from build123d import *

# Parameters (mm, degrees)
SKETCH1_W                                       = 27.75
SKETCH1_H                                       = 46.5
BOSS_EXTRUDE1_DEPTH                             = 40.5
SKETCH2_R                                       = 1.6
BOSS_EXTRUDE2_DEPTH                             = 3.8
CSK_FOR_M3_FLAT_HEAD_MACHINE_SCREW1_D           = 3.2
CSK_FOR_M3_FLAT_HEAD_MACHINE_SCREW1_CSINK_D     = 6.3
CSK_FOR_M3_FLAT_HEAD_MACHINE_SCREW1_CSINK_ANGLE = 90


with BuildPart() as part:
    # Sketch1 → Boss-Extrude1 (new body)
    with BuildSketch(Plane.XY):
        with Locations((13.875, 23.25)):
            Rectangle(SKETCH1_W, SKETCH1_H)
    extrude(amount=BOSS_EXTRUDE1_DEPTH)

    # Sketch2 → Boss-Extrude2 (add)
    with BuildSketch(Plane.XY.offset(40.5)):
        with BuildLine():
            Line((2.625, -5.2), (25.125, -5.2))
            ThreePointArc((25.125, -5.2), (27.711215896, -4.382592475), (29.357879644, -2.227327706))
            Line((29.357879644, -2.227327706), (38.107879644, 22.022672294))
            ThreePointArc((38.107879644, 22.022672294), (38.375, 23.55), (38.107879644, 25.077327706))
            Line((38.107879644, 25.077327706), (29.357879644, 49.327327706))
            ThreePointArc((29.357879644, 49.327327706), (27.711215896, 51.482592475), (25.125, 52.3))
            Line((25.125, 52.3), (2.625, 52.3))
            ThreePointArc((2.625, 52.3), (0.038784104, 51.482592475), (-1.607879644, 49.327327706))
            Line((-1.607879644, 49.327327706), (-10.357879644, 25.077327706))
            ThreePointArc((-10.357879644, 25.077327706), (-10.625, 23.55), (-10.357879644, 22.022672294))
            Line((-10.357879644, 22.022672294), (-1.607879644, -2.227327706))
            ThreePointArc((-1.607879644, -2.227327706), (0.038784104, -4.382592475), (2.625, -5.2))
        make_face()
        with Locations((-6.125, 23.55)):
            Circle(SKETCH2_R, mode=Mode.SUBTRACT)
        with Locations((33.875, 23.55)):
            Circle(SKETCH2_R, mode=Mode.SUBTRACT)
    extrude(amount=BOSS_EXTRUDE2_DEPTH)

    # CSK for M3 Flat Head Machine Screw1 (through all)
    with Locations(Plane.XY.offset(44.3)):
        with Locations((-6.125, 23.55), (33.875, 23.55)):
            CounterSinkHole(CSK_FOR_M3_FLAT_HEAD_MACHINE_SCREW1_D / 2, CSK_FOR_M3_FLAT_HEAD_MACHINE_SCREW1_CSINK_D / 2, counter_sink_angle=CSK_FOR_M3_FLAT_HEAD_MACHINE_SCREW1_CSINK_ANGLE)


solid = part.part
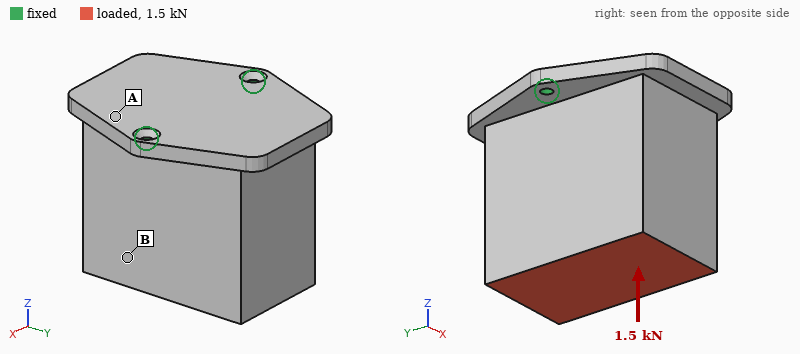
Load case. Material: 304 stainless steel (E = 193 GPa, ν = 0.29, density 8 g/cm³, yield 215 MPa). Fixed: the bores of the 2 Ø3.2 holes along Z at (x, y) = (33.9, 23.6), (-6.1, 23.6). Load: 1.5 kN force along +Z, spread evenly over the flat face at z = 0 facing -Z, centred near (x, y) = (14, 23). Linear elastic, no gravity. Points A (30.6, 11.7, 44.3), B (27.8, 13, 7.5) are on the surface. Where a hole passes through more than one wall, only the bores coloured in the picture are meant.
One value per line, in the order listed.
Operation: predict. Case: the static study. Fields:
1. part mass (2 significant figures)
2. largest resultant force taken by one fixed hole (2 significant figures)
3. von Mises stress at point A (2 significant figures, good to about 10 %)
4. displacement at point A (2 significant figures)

490 g
750 N
21 MPa
6.0 µm
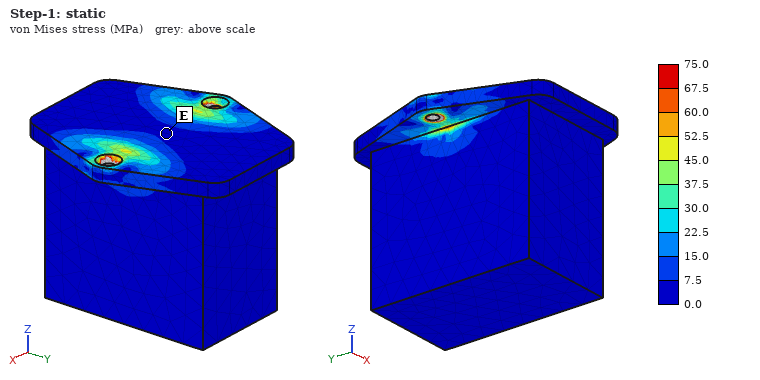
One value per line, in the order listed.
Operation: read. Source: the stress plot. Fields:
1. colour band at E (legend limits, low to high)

0.0 to 7.5 MPa
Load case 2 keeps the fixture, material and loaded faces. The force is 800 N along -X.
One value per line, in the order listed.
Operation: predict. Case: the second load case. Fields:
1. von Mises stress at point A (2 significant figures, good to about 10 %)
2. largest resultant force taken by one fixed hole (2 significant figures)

30 MPa
1.0 kN
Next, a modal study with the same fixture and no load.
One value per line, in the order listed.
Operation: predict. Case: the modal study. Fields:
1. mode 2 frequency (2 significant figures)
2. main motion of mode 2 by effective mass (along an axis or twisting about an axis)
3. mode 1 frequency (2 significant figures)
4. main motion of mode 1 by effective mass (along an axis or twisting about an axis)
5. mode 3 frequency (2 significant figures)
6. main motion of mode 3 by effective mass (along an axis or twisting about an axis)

2600 Hz
along X
590 Hz
along Y
3700 Hz
along Z
